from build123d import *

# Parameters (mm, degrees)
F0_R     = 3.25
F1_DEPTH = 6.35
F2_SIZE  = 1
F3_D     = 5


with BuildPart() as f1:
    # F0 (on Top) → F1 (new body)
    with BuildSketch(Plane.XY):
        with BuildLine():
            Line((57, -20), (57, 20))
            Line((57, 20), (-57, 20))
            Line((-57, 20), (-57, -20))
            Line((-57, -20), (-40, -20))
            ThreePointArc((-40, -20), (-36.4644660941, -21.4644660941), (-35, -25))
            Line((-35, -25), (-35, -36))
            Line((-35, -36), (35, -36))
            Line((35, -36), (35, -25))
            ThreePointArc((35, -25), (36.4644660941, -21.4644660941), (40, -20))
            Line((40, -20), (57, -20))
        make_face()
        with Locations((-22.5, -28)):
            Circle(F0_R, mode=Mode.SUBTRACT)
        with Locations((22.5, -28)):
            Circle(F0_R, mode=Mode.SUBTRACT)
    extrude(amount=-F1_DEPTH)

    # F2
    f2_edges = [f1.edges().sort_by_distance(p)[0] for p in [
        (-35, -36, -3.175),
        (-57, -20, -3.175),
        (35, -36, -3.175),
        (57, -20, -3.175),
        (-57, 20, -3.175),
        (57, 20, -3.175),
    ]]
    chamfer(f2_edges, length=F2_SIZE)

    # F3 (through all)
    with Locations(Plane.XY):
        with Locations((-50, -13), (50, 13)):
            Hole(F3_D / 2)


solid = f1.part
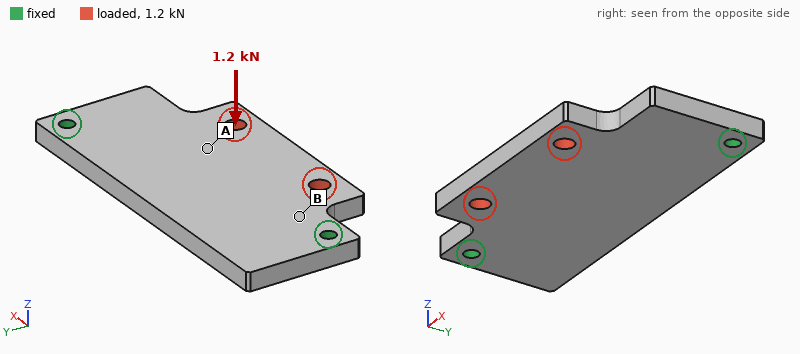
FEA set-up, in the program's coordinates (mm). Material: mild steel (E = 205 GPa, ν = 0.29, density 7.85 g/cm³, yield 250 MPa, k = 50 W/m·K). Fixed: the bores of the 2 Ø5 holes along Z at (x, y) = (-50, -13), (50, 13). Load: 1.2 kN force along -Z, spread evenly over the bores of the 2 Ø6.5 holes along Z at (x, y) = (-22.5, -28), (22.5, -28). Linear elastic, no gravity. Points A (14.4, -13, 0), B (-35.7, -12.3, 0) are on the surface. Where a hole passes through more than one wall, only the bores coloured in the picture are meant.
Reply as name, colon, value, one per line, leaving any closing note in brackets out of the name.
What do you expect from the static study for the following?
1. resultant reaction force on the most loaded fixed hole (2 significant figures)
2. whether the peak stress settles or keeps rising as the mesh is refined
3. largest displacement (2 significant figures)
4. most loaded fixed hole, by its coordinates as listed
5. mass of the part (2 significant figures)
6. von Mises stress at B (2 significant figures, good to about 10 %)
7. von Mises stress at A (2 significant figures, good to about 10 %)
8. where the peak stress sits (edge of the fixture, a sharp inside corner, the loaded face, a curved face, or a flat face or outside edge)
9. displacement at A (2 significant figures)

resultant reaction force on the most loaded fixed hole: 700 N
whether the peak stress settles or keeps rising as the mesh is refined: keeps rising
largest displacement: 0.14 mm
most loaded fixed hole, by its coordinates as listed: (-50, -13)
mass of the part: 280 g
von Mises stress at B: 78 MPa
von Mises stress at A: 36 MPa
where the peak stress sits: edge of the fixture
displacement at A: 0.067 mm
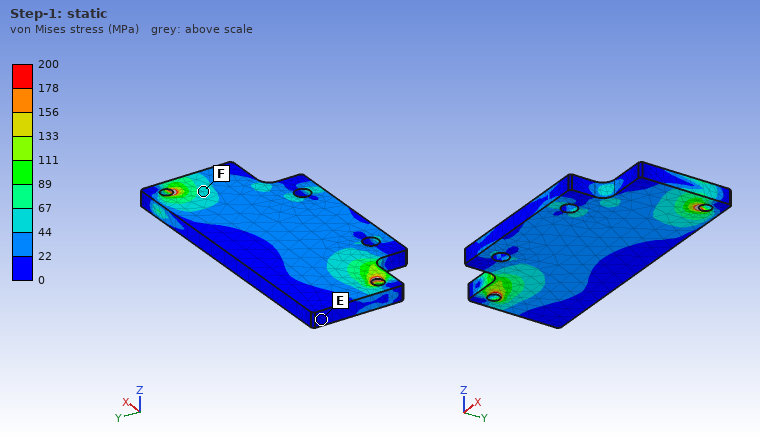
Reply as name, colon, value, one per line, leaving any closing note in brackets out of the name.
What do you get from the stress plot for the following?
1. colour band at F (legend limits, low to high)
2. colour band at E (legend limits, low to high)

colour band at F: 44 to 67 MPa
colour band at E: 0 to 22 MPa
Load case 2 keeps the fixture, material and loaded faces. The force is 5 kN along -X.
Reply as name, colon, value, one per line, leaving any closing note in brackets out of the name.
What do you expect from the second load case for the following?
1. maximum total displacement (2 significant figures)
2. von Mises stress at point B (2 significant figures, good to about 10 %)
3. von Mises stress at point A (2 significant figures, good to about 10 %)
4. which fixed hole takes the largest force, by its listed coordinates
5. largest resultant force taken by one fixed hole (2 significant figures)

maximum total displacement: 8.3 µm
von Mises stress at point B: 22 MPa
von Mises stress at point A: 11 MPa
which fixed hole takes the largest force, by its listed coordinates: (-50, -13)
largest resultant force taken by one fixed hole: 3.2 kN
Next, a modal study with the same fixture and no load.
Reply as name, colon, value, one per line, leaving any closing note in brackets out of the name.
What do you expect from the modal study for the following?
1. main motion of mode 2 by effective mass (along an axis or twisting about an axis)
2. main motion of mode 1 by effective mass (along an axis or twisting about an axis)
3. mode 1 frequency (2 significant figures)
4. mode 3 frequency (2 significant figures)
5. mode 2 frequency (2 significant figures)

main motion of mode 2 by effective mass: along Z
main motion of mode 1 by effective mass: along Z
mode 1 frequency: 1900 Hz
mode 3 frequency: 5100 Hz
mode 2 frequency: 2800 Hz
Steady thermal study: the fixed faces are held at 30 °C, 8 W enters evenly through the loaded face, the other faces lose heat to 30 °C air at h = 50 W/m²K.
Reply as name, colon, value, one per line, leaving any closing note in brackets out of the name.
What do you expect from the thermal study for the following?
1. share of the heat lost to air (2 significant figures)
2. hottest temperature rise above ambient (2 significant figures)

share of the heat lost to air: 48 %
hottest temperature rise above ambient: 14 K
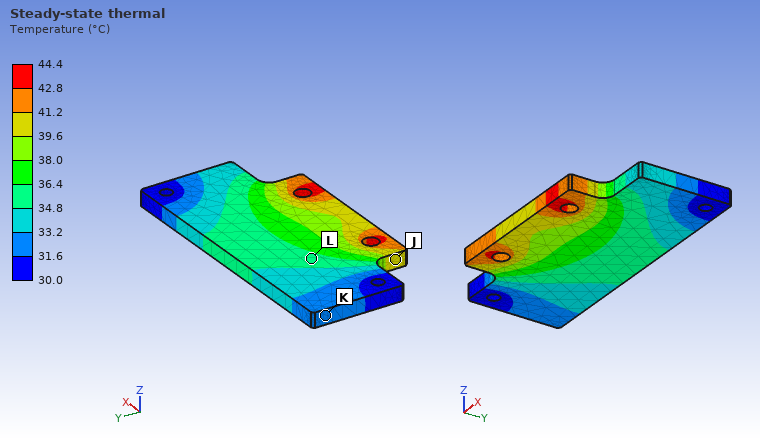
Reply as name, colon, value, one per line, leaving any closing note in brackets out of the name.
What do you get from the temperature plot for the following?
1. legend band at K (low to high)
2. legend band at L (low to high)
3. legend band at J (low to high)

legend band at K: 31.6 to 33.2 °C
legend band at L: 34.8 to 36.4 °C
legend band at J: 39.6 to 41.2 °C
